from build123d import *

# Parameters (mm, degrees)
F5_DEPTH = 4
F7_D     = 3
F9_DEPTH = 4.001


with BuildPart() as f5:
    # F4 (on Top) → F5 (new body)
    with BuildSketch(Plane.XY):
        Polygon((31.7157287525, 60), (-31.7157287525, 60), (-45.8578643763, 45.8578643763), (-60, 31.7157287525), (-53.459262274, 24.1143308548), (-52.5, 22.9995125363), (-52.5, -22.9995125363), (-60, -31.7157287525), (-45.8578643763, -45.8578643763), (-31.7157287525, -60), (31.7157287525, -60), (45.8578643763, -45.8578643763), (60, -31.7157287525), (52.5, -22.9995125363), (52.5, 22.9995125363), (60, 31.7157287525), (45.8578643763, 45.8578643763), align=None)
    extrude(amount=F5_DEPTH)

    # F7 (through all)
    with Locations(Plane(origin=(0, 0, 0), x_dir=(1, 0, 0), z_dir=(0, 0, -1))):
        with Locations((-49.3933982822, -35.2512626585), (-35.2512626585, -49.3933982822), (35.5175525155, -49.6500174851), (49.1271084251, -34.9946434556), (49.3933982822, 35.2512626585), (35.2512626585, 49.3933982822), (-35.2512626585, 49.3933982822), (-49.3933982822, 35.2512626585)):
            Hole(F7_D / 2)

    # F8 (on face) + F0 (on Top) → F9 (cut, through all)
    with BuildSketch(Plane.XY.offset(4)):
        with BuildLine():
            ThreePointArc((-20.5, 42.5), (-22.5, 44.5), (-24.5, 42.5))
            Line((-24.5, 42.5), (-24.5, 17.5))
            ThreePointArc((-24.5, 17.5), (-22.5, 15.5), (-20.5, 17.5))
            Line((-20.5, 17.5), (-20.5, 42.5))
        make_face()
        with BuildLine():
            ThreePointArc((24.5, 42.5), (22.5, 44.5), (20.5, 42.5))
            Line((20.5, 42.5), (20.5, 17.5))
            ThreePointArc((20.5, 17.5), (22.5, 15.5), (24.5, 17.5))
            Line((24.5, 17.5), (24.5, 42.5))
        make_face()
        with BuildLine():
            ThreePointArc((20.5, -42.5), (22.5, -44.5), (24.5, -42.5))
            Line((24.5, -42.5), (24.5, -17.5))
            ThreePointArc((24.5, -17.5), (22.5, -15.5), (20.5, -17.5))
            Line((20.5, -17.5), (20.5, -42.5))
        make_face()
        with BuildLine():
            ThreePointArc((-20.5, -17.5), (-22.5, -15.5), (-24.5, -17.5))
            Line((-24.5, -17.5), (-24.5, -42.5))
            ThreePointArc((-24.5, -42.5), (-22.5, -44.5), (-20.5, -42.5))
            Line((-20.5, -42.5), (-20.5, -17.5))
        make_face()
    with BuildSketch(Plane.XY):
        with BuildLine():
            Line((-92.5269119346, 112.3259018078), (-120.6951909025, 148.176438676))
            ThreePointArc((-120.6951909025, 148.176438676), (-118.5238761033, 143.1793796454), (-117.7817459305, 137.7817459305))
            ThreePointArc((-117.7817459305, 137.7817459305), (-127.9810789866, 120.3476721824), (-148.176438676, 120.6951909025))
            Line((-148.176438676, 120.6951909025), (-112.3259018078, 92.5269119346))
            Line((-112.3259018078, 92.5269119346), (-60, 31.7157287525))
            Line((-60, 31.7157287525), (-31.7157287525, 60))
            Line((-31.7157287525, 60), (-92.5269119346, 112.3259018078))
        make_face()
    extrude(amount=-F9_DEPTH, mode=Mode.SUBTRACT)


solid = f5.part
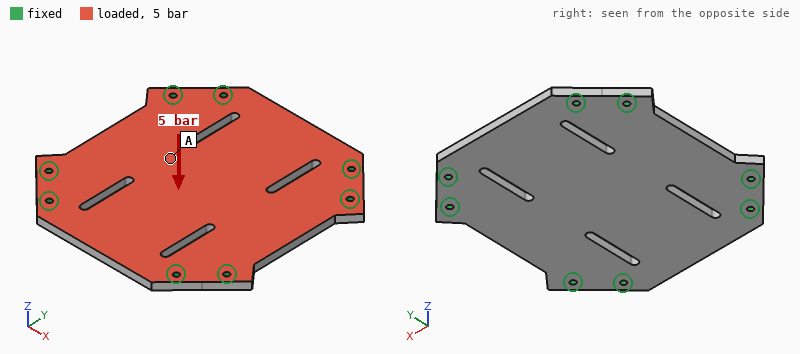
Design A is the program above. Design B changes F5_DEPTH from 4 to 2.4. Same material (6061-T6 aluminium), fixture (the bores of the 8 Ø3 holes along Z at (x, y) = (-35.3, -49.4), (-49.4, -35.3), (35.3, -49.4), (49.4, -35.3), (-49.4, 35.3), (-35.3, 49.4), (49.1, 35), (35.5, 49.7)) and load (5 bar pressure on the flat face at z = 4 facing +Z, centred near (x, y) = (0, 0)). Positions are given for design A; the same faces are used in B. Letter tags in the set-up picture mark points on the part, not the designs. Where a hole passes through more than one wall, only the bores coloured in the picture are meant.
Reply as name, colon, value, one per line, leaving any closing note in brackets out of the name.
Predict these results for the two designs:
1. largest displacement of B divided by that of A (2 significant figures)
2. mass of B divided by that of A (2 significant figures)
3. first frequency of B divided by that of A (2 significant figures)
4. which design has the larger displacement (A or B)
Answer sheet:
largest displacement of B divided by that of A: 4.3
mass of B divided by that of A: 0.60
first frequency of B divided by that of A: 0.62
which design has the larger displacement: B
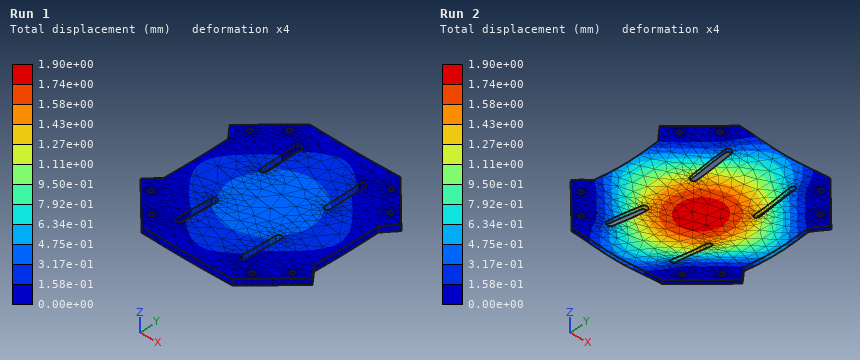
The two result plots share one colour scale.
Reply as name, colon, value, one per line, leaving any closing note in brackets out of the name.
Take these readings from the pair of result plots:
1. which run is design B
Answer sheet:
which run is design B: Run 2
